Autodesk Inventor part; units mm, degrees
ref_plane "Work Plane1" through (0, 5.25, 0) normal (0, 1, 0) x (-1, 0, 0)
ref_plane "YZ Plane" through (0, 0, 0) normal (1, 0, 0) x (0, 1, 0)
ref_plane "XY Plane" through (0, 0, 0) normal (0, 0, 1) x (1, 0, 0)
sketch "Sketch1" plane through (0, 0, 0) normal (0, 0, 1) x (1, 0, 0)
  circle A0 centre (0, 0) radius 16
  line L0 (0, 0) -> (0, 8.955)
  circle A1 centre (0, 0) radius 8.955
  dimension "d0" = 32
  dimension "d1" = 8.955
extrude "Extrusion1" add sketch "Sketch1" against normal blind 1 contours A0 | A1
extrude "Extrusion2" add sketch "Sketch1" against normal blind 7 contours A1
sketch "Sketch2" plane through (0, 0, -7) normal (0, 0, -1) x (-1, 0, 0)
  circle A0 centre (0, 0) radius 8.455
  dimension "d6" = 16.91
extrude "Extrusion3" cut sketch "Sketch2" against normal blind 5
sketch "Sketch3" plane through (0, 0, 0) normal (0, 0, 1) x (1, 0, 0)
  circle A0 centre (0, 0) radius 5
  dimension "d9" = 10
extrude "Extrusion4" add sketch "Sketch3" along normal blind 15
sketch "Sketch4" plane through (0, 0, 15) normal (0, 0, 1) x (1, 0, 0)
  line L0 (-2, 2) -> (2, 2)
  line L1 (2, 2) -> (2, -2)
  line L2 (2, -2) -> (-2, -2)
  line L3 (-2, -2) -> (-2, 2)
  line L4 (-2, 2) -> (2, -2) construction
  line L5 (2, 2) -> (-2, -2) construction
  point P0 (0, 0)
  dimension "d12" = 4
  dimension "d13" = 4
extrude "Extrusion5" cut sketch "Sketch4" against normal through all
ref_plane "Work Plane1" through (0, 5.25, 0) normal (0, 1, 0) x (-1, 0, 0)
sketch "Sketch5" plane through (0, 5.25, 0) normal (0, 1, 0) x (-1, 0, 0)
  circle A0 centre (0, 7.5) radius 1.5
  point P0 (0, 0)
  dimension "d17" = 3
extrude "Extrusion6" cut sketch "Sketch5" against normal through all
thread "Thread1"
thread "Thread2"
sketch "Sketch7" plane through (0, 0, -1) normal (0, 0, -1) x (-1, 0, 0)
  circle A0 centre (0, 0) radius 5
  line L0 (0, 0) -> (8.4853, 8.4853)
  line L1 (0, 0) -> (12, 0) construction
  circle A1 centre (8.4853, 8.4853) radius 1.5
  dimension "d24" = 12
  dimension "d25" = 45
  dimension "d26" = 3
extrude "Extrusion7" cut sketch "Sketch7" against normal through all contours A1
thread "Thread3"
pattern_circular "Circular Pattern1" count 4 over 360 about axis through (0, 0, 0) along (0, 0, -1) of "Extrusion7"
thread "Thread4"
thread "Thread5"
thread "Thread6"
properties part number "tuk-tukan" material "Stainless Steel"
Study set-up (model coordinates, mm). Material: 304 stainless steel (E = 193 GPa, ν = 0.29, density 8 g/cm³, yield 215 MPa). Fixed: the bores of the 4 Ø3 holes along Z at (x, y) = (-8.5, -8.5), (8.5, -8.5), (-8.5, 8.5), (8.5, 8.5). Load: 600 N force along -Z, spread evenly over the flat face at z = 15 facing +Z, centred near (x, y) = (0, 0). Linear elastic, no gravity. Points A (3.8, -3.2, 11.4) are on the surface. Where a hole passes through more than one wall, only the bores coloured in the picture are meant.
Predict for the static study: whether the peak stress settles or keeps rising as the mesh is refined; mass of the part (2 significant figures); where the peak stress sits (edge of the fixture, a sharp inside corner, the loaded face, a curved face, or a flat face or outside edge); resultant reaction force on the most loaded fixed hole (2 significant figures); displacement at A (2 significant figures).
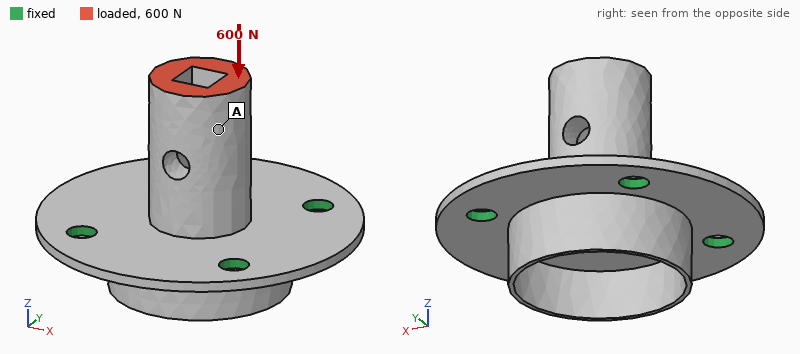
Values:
keeps rising
16 g
edge of the fixture
180 N
8.4 µm
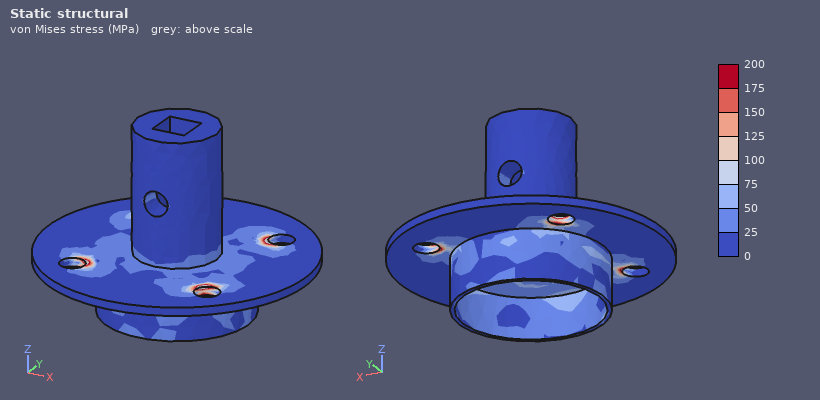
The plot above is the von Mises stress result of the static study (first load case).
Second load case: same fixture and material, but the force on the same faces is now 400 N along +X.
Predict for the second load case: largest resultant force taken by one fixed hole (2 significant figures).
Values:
240 N
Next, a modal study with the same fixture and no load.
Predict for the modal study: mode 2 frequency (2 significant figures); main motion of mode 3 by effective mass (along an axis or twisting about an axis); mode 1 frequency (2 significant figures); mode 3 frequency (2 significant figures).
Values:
9600 Hz
along Z
9500 Hz
14 kHz
